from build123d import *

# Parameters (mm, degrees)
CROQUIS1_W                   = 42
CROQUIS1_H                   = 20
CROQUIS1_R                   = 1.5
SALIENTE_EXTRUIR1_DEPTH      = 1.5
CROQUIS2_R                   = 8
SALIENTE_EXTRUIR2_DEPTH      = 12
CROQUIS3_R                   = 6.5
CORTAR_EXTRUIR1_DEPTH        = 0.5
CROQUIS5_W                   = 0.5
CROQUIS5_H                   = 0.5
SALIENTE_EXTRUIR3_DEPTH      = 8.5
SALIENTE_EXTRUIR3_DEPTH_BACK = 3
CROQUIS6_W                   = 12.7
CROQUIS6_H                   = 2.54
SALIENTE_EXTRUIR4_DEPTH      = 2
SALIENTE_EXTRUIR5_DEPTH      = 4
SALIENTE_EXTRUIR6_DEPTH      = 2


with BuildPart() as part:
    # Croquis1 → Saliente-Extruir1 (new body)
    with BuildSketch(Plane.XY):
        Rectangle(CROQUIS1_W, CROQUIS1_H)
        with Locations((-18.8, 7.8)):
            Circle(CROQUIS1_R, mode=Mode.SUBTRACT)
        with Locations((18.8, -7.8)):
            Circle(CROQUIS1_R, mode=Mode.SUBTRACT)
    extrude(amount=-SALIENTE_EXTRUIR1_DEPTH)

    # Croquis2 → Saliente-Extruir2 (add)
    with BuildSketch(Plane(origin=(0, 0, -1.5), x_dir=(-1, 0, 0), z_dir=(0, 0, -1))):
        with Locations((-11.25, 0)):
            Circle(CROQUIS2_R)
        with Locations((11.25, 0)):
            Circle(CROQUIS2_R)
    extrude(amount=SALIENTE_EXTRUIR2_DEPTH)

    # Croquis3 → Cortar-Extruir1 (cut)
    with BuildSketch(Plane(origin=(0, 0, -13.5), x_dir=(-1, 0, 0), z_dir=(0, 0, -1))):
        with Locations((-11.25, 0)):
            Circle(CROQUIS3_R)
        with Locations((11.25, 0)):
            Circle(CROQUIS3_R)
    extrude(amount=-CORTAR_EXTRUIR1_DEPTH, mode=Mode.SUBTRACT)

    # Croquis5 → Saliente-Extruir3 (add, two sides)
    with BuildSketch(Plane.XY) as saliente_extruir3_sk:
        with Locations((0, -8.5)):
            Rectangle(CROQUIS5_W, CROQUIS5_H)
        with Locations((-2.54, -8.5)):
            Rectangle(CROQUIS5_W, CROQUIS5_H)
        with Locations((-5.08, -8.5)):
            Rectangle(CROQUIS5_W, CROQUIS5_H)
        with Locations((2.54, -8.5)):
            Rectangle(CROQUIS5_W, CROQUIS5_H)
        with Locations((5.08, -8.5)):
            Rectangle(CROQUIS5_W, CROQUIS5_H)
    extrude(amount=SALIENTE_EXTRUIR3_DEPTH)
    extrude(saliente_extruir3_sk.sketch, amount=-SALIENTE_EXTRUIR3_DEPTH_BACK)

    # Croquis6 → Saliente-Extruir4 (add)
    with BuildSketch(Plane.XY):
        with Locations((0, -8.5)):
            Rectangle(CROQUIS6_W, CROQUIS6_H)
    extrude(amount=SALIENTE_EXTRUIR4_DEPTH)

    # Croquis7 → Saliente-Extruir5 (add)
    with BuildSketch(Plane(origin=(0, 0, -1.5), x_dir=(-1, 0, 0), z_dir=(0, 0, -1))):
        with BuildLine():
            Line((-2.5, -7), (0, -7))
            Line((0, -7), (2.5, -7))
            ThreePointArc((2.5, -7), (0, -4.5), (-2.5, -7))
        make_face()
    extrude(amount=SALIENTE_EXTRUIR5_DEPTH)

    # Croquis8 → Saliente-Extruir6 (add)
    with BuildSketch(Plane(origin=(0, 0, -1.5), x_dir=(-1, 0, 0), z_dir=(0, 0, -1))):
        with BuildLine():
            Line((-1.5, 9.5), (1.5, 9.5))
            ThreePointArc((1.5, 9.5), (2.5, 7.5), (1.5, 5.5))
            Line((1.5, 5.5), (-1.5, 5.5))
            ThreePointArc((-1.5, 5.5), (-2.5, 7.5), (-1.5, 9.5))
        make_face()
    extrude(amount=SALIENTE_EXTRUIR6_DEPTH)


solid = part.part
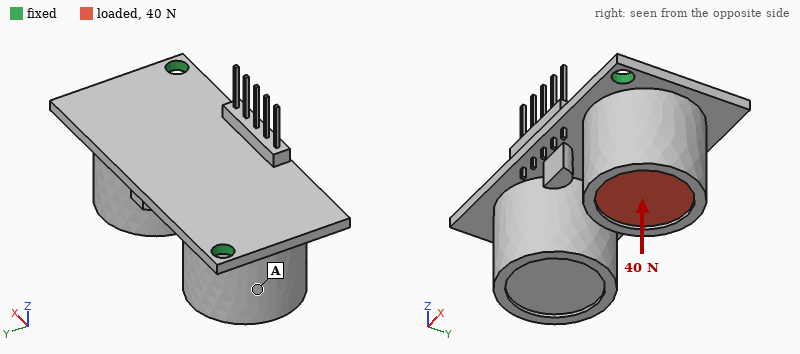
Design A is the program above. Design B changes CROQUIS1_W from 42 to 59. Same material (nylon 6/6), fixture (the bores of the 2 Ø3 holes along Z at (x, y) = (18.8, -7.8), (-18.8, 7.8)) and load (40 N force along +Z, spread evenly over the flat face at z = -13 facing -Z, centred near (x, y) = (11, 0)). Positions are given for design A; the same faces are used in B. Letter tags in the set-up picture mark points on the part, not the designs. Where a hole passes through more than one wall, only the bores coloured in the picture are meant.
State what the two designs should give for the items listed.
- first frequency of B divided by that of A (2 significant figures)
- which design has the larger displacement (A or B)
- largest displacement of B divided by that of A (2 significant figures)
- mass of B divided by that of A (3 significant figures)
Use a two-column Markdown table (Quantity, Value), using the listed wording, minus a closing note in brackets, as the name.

| Quantity | Value |
|---|---|
| first frequency of B divided by that of A | 1.0 |
| which design has the larger displacement | A |
| largest displacement of B divided by that of A | 0.91 |
| mass of B divided by that of A | 1.08 |
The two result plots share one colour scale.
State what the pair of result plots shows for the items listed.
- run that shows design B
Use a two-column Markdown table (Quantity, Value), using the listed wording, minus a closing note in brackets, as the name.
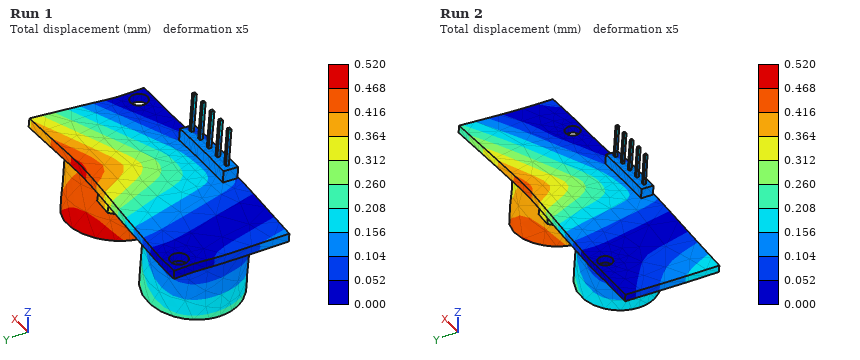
| Quantity | Value |
|---|---|
| run that shows design B | Run 2 |
